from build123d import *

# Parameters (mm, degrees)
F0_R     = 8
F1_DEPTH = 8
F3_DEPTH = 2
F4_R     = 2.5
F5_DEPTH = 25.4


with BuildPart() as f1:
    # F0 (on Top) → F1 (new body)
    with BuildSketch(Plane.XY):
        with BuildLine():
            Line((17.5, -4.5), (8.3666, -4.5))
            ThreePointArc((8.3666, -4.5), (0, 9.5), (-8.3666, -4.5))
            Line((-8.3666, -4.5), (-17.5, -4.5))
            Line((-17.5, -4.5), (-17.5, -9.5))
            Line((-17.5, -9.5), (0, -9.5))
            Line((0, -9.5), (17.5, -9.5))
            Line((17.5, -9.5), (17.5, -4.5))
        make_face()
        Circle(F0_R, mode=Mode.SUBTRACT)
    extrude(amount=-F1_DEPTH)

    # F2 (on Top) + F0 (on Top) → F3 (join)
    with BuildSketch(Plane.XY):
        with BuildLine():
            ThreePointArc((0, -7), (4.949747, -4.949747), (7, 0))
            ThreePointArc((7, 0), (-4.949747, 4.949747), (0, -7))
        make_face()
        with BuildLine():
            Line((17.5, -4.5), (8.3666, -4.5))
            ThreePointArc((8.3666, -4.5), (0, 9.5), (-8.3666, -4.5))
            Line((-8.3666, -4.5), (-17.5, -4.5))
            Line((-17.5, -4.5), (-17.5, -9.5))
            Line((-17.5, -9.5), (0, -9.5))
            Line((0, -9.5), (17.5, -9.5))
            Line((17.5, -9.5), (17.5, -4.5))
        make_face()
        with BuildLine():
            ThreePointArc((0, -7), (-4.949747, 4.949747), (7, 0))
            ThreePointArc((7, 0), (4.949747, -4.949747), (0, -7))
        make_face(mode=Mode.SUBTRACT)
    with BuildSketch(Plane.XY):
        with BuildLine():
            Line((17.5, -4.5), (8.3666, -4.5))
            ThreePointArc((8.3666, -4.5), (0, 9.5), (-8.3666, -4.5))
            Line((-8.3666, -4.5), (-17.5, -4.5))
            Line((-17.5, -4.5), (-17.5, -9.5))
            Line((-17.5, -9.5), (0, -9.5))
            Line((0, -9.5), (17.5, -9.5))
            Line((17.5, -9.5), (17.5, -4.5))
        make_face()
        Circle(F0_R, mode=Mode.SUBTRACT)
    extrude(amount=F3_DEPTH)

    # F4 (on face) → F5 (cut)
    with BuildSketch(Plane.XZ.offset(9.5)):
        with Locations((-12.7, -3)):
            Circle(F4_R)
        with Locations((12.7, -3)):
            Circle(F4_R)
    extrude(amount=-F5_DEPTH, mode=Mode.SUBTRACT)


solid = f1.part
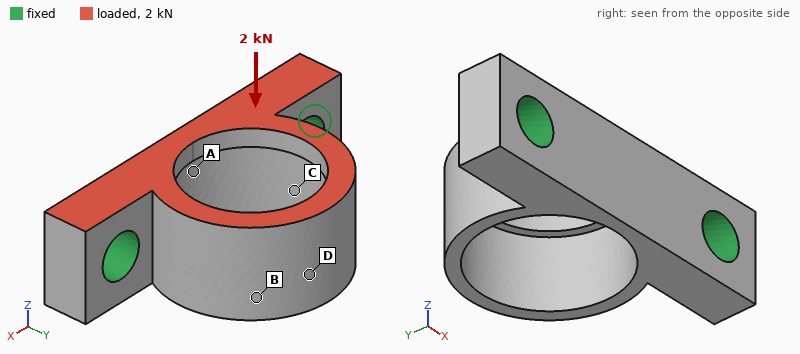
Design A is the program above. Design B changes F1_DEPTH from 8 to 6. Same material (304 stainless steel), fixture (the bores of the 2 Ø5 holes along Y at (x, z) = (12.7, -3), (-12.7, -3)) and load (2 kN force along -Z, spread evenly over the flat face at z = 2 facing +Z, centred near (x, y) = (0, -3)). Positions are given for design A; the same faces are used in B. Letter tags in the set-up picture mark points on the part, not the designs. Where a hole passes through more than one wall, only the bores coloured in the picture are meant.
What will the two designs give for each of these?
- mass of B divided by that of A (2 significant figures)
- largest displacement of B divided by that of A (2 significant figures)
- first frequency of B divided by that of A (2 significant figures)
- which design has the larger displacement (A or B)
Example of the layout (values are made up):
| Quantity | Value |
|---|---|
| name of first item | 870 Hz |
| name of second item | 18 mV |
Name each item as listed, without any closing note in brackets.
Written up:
| Quantity | Value |
|---|---|
| mass of B divided by that of A | 0.79 |
| largest displacement of B divided by that of A | 1.5 |
| first frequency of B divided by that of A | 1.0 |
| which design has the larger displacement | B |
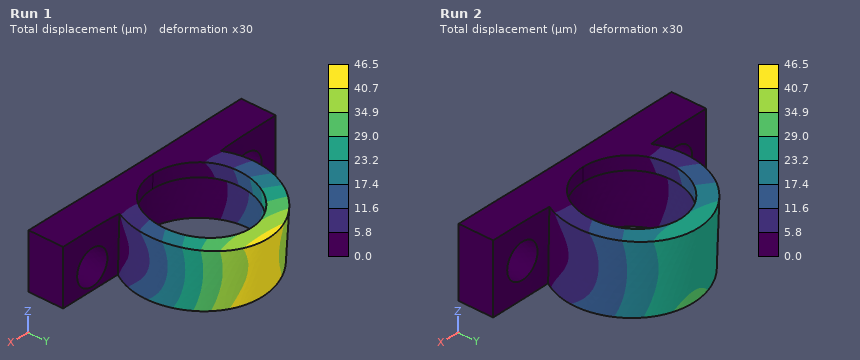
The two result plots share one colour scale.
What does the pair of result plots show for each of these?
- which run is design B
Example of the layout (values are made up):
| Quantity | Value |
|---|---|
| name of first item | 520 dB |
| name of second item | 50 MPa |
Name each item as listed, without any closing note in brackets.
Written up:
| Quantity | Value |
|---|---|
| which run is design B | Run 1 |
